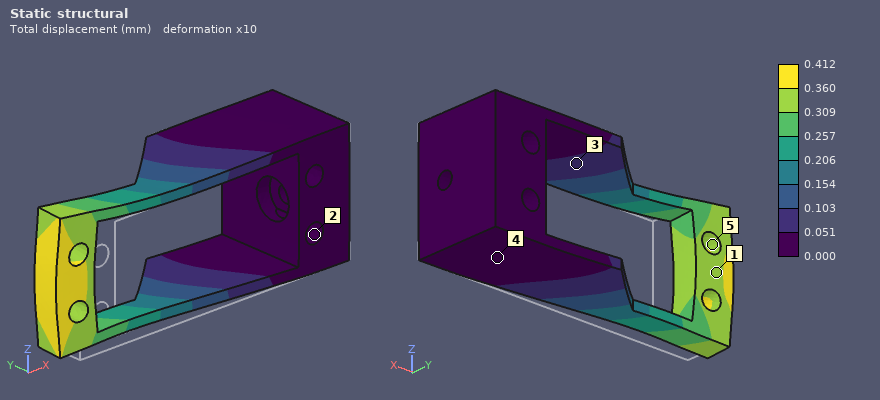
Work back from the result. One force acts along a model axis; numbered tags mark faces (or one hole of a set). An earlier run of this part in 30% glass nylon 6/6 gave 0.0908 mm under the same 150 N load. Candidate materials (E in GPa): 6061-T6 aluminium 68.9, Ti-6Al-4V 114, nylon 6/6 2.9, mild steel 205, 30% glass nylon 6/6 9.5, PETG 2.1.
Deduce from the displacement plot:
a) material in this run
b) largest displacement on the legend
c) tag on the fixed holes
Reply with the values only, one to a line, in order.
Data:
PETG
0.412 mm
2
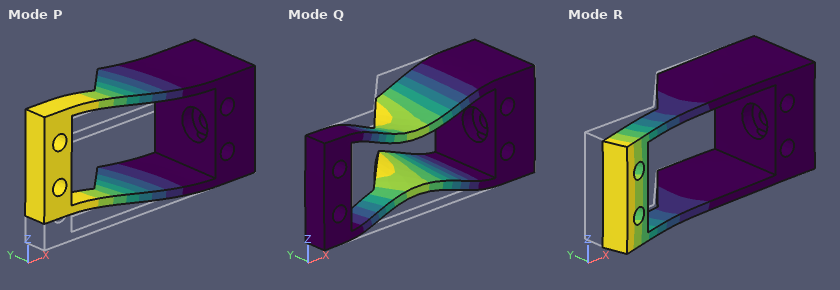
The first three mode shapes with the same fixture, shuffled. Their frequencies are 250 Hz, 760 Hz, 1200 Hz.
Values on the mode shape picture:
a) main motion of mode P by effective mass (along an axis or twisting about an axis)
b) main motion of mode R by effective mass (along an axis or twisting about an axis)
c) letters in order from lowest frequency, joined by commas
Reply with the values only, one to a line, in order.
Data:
along Z
along Y
P, R, Q
